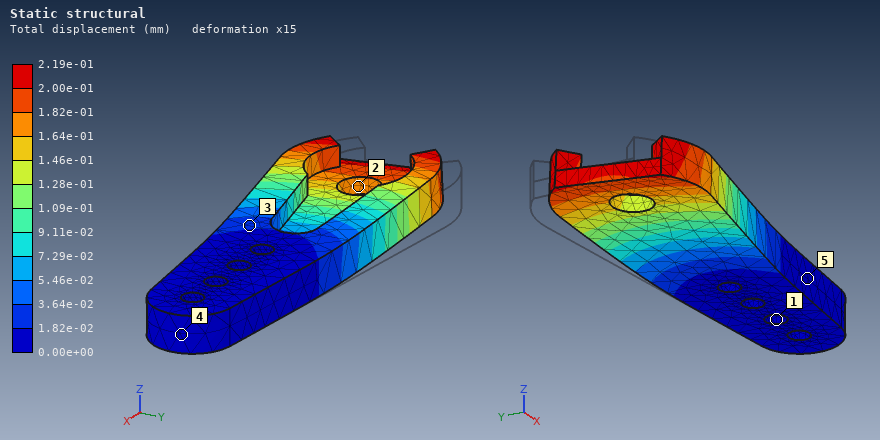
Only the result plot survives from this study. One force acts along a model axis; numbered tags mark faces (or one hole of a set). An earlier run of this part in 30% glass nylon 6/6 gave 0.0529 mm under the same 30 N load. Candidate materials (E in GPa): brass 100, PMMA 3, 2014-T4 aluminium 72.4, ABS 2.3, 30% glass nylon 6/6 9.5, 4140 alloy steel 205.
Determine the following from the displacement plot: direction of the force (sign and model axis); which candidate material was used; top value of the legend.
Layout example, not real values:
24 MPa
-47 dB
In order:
-Y
ABS
2.19e-01 mm
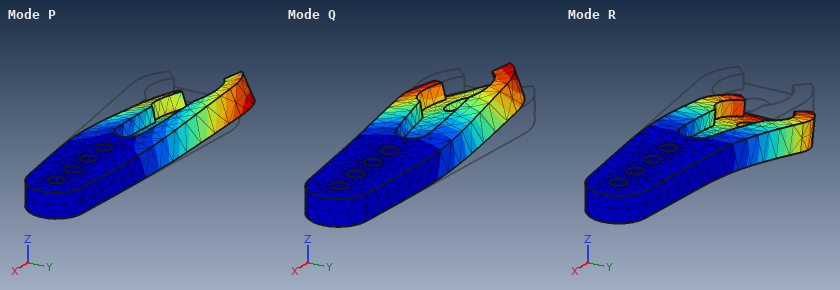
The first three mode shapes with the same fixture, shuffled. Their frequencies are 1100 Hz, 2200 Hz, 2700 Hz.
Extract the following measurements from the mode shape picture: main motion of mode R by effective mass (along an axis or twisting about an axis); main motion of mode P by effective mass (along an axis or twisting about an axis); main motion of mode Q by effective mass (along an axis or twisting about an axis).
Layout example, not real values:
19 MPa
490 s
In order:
along Z
along Y
along Y
